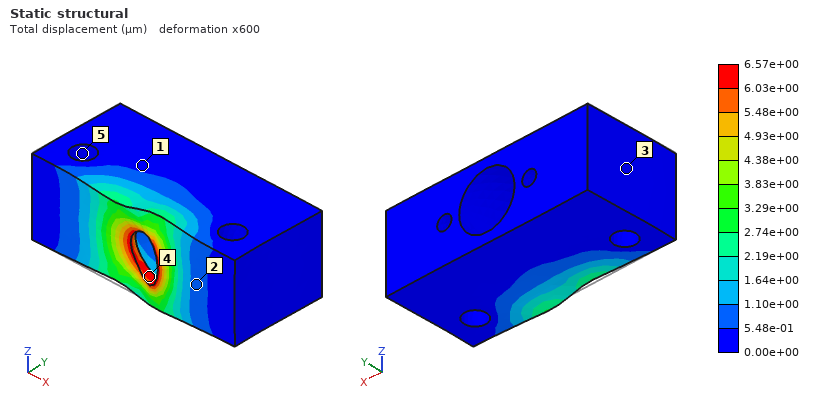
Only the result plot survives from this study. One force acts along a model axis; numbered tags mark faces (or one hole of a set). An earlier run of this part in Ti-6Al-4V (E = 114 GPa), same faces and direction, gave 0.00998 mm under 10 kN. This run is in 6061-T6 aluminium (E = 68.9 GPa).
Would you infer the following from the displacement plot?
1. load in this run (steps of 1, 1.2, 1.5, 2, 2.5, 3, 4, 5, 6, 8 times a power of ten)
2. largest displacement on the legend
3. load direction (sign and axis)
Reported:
4 kN
6.57e+00 µm
+X
